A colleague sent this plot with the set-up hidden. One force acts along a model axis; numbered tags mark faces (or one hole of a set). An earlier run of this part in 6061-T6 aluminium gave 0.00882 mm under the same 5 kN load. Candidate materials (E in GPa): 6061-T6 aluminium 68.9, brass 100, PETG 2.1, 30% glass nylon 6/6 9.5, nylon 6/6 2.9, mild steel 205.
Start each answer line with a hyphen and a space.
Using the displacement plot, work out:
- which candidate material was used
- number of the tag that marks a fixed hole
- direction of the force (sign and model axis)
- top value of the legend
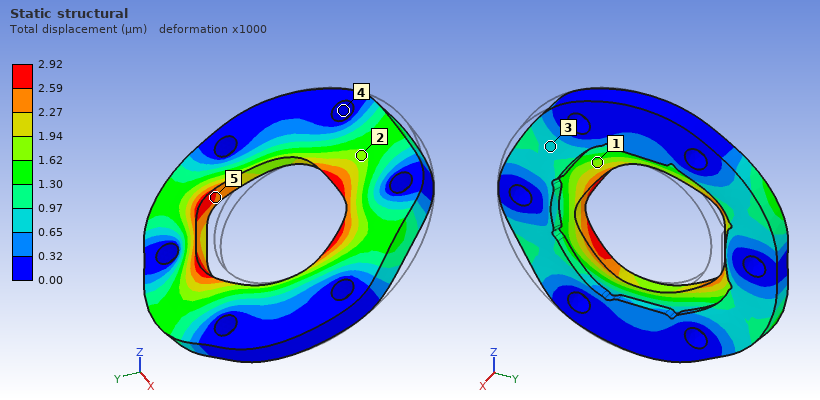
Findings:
- mild steel
- 4
- +Y
- 2.92 µm
